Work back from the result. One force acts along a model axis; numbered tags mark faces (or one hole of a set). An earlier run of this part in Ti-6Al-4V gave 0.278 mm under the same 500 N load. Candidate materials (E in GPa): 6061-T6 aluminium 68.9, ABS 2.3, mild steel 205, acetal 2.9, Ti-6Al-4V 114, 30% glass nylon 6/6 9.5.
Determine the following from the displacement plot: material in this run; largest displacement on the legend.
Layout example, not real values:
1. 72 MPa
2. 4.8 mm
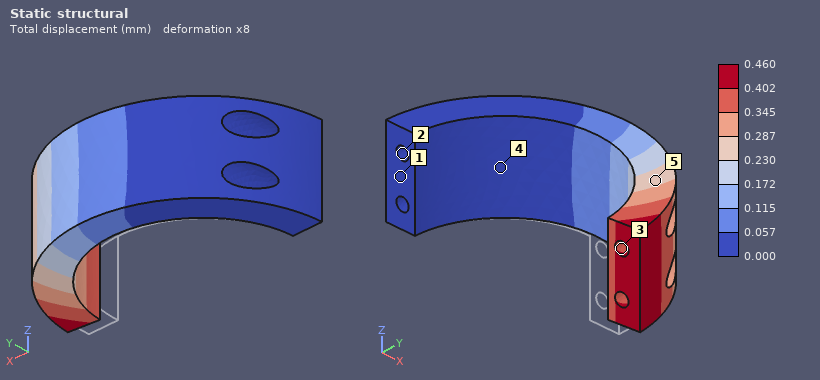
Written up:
1. 6061-T6 aluminium
2. 0.460 mm
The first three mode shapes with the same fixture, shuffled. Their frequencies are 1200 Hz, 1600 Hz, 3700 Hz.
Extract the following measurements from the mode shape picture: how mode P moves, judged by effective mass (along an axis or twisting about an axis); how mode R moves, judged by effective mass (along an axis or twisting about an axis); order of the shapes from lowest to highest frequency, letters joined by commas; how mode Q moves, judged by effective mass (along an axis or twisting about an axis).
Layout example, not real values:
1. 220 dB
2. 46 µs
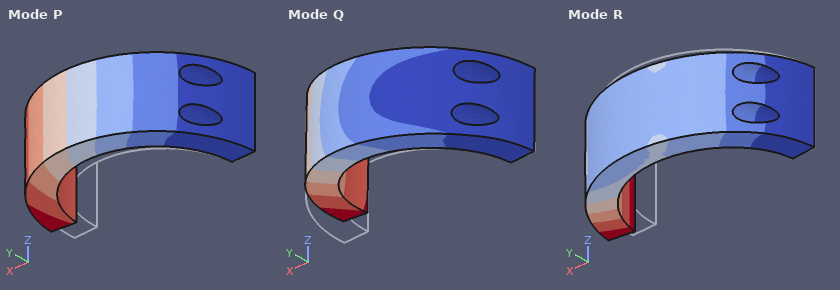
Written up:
1. along Y
2. along X
3. P, Q, R
4. along Z
